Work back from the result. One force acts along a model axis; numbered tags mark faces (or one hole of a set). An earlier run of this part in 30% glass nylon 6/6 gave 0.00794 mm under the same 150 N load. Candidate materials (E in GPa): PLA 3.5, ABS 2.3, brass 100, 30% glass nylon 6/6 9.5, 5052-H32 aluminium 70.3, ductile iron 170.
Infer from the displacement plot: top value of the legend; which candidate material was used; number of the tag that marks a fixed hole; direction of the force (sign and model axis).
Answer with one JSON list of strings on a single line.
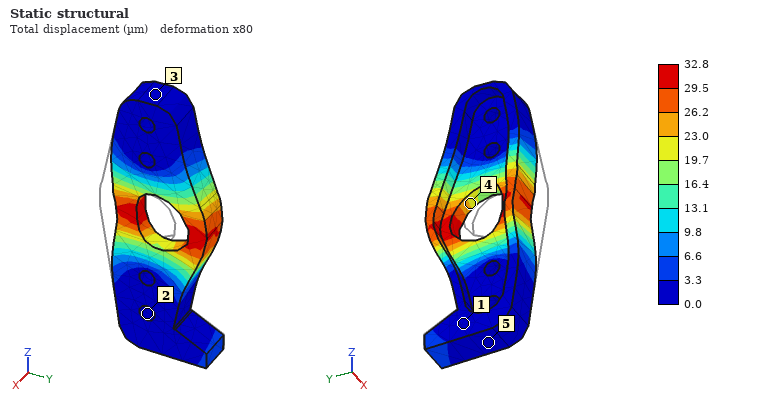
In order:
["32.8 µm", "ABS", "2", "+Y"]
